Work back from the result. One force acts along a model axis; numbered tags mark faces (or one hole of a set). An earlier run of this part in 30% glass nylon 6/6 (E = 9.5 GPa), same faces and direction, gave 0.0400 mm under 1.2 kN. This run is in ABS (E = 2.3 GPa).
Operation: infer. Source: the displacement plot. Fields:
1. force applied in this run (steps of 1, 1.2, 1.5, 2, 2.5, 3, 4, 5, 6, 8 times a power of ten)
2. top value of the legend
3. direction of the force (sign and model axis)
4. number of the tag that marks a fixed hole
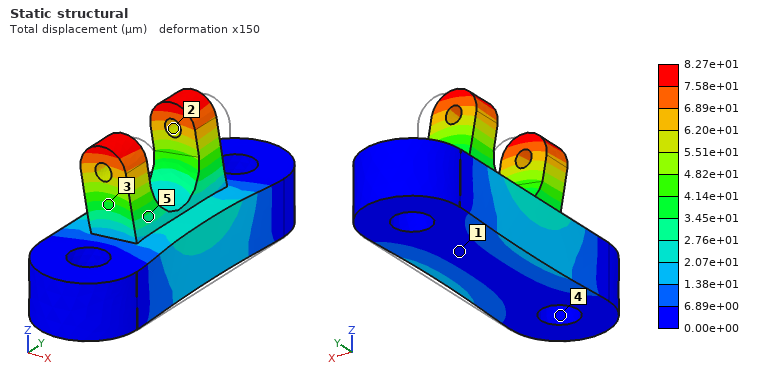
600 N
8.27e+01 µm
-X
4
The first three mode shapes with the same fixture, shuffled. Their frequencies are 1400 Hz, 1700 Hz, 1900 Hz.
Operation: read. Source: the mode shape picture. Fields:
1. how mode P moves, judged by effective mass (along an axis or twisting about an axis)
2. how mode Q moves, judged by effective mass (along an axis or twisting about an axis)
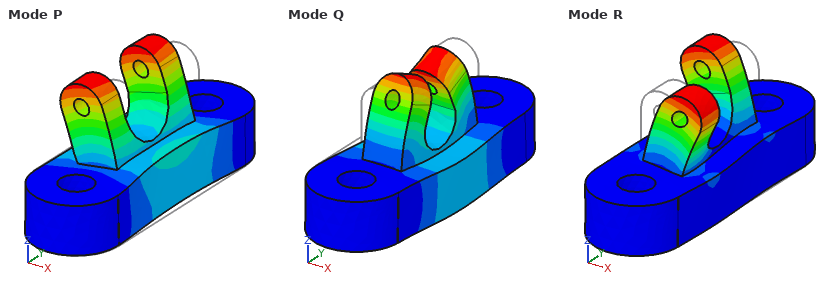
along X
along Z
